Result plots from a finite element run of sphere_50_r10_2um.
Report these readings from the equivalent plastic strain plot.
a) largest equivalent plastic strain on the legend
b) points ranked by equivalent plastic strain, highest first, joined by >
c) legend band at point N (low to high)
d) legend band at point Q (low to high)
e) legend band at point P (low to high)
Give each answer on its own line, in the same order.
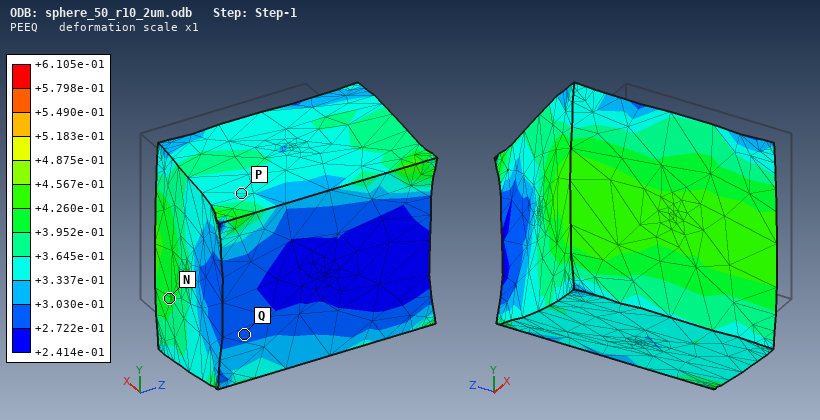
+6.105e-01
N > P > Q
+3.952e-01 to +4.260e-01
+2.722e-01 to +3.030e-01
+3.337e-01 to +3.645e-01
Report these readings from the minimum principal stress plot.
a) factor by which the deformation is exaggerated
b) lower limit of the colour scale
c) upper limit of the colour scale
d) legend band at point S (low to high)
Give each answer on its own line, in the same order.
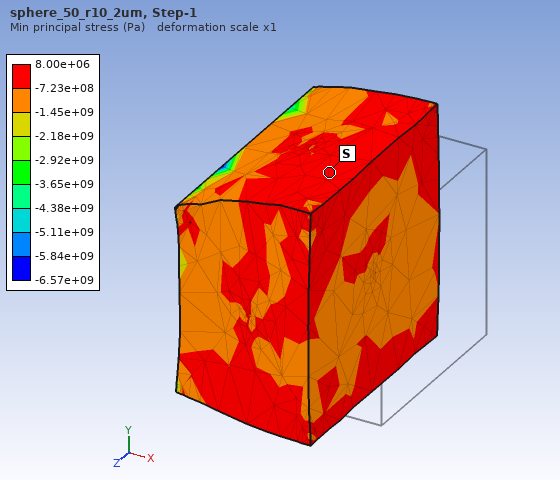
1
-6.57e+09 Pa
8.00e+06 Pa
-7.23e+08 to 8.00e+06 Pa
